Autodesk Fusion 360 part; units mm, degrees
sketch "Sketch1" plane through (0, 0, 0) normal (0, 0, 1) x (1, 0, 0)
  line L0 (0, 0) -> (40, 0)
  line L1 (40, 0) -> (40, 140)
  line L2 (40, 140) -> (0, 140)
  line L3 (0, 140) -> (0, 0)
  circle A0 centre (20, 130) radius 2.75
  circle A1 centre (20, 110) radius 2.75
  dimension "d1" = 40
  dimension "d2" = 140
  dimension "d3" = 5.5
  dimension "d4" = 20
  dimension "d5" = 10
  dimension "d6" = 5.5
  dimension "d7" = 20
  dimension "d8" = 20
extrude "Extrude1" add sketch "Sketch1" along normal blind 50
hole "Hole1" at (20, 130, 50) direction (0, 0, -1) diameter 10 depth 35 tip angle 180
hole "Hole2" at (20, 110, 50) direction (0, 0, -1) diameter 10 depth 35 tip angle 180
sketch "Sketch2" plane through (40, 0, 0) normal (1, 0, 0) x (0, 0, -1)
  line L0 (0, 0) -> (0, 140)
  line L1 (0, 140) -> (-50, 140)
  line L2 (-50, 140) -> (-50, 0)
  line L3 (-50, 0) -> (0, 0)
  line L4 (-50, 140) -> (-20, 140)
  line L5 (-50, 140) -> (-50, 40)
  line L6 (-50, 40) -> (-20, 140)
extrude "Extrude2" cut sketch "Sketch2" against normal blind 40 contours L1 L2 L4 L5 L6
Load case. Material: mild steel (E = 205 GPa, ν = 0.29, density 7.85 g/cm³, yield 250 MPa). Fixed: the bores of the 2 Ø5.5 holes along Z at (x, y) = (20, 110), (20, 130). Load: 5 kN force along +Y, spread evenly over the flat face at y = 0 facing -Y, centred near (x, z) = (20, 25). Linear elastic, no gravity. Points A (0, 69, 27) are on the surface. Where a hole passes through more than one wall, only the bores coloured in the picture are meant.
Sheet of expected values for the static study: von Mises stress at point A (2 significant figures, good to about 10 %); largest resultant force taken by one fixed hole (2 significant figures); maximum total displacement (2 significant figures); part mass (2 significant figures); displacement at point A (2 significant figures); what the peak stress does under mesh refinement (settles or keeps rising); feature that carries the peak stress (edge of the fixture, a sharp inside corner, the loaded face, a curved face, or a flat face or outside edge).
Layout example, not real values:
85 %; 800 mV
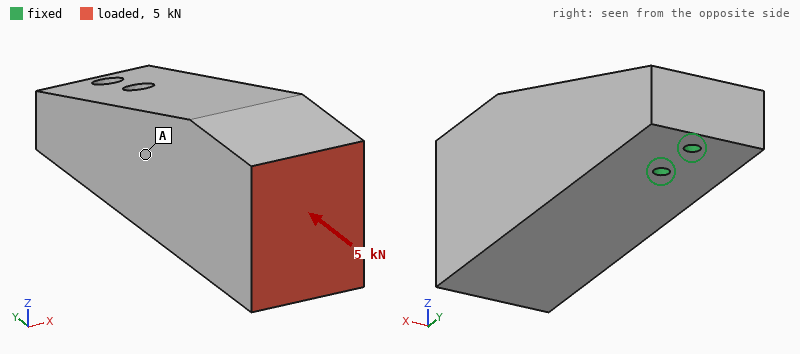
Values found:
4.1 MPa; 3.8 kN; 22 µm; 1.7 kg; 8.1 µm; keeps rising; edge of the fixture
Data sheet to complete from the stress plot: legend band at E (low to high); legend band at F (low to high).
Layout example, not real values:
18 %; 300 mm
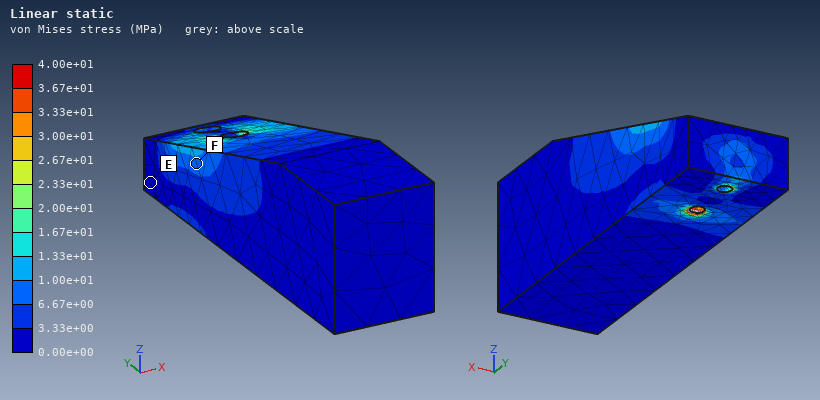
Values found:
0.00e+00 to 3.33e+00 MPa; 6.67e+00 to 1.00e+01 MPa
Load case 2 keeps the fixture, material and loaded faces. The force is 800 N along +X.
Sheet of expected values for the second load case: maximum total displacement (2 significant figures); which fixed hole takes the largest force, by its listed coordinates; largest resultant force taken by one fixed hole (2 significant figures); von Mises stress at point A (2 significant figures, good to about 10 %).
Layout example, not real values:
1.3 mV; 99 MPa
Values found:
24 µm; (20, 110); 4.3 kN; 5.0 MPa
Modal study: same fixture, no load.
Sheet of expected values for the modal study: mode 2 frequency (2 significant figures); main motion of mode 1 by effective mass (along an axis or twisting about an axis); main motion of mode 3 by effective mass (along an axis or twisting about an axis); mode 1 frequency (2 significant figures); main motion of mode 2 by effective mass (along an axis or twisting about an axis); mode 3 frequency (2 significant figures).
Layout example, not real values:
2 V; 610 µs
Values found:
1300 Hz; along Z; twisting about Y; 1100 Hz; along X; 3500 Hz
